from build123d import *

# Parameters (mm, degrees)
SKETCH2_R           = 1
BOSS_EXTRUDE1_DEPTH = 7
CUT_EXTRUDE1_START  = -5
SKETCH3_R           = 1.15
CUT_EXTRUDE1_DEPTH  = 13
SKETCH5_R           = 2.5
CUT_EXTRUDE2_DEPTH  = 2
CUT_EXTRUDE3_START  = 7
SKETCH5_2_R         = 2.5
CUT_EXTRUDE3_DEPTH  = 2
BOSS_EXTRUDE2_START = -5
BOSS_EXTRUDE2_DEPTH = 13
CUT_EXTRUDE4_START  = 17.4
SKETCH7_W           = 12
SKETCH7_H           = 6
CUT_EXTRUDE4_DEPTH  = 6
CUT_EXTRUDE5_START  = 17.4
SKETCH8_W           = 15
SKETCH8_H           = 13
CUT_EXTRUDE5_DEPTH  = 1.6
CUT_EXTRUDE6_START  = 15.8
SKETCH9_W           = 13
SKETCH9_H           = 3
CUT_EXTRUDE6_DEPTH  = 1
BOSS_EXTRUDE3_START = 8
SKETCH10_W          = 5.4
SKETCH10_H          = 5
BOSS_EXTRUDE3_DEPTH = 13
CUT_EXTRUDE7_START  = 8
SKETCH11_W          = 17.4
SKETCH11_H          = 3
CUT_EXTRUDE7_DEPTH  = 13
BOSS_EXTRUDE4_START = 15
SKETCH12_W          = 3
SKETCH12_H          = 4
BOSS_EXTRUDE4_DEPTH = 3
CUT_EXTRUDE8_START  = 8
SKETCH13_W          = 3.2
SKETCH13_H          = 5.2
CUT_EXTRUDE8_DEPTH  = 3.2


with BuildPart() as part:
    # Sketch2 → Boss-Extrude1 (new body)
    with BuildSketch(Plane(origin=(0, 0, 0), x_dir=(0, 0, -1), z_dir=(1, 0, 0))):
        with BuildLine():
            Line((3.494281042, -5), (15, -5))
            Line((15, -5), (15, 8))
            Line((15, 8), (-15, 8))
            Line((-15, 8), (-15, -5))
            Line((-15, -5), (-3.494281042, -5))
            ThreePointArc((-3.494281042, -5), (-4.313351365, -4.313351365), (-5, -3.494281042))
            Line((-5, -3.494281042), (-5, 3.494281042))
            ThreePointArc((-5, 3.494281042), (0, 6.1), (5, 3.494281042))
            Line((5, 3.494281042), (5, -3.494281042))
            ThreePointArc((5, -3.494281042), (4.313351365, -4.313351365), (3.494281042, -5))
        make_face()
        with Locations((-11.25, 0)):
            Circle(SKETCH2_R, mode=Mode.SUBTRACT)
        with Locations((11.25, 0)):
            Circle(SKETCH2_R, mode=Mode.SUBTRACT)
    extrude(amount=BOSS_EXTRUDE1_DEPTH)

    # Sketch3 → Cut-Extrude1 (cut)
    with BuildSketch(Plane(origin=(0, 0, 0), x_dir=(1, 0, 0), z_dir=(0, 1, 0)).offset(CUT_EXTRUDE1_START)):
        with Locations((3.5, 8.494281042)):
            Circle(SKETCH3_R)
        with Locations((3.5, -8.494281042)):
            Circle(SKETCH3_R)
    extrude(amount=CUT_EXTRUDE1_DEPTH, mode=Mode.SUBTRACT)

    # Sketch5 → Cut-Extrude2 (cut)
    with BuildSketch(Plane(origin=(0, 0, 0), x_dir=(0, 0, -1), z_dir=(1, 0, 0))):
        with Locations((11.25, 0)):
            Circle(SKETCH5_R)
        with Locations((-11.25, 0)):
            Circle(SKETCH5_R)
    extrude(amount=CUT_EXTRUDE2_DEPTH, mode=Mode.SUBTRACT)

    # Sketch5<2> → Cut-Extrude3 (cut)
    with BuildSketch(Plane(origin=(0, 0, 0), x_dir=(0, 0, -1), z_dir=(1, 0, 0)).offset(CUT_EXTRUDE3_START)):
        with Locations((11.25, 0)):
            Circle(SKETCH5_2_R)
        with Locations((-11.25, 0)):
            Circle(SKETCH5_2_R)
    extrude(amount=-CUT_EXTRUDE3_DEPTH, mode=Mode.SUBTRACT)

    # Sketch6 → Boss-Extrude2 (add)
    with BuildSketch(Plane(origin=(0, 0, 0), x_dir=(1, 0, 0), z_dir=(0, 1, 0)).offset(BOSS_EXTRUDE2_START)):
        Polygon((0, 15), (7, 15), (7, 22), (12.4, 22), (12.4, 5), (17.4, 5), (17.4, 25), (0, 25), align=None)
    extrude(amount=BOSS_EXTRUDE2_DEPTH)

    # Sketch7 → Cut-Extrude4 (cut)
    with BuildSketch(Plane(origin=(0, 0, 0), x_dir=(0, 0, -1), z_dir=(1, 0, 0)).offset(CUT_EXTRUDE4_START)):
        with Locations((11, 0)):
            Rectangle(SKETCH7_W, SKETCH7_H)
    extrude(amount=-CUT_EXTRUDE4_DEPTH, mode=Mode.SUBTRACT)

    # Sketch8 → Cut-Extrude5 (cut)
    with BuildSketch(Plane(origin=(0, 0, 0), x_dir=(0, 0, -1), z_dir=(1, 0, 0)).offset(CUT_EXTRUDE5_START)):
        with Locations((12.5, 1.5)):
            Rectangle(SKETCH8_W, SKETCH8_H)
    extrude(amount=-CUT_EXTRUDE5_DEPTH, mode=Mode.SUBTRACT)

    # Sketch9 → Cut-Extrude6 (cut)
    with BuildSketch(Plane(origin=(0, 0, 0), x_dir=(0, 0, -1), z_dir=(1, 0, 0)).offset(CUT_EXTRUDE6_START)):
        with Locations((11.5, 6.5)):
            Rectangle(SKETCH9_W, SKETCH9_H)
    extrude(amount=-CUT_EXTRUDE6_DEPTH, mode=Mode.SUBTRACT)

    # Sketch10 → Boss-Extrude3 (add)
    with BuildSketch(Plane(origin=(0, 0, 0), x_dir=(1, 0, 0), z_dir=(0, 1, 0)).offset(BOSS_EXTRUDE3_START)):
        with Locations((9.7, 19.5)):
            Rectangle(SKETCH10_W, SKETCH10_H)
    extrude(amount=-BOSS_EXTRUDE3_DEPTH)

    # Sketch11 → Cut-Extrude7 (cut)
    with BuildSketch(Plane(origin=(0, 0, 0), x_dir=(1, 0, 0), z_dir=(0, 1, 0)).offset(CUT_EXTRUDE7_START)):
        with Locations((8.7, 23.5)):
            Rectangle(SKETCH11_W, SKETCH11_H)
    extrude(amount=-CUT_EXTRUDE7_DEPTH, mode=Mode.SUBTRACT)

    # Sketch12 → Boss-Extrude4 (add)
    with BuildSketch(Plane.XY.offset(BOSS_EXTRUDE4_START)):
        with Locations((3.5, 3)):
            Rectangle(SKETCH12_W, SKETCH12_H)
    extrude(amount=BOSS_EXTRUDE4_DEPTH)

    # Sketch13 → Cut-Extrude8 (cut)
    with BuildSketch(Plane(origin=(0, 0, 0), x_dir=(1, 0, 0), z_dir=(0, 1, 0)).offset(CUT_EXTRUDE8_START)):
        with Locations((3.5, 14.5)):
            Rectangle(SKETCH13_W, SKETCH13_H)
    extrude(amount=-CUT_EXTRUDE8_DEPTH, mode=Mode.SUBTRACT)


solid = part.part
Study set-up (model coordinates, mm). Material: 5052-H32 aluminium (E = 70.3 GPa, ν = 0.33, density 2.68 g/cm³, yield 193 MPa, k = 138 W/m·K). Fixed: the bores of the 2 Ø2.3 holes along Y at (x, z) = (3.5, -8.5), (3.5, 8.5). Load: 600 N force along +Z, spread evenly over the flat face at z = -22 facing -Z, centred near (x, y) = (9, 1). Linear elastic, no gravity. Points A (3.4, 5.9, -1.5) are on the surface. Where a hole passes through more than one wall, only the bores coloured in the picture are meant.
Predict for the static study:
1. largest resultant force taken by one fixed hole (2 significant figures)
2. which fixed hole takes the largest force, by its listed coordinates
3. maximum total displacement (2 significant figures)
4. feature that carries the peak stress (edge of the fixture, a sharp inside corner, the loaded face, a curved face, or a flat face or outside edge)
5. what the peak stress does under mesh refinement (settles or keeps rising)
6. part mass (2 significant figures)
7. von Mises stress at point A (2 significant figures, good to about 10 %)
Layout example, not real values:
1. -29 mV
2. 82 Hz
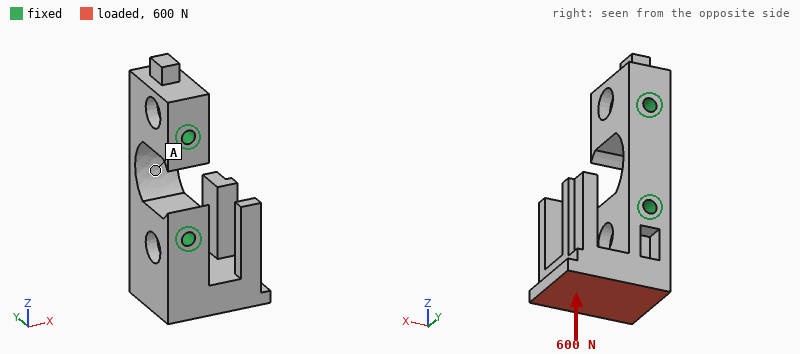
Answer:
1. 590 N
2. (3.5, -8.5)
3. 47 µm
4. edge of the fixture
5. keeps rising
6. 8.6 g
7. 9.0 MPa
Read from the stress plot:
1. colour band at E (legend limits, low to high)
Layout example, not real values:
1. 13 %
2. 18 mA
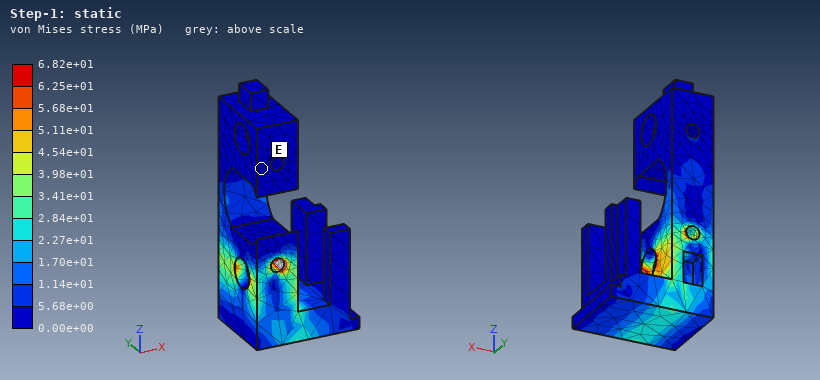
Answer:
1. 0.00e+00 to 5.68e+00 MPa
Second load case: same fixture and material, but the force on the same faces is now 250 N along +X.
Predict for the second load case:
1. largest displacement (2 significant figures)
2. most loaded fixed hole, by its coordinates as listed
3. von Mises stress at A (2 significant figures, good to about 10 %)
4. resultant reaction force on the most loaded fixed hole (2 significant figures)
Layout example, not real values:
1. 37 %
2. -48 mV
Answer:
1. 33 µm
2. (3.5, -8.5)
3. 9.1 MPa
4. 290 N
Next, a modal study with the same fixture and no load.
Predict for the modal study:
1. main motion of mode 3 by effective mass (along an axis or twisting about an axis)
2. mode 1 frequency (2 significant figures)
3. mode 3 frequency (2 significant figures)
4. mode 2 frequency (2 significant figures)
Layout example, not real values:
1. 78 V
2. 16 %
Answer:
1. along X
2. 9000 Hz
3. 12 kHz
4. 9100 Hz
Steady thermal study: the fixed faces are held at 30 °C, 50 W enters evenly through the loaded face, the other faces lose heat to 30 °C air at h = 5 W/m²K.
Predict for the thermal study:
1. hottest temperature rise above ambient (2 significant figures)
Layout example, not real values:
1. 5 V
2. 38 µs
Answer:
1. 77 K
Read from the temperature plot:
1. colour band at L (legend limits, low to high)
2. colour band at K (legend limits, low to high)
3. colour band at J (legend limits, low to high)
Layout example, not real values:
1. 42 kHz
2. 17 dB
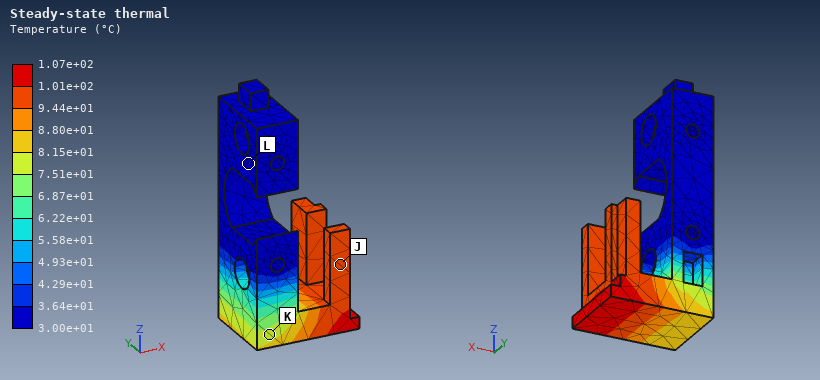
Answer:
1. 3.00e+01 to 3.64e+01 °C
2. 7.51e+01 to 8.15e+01 °C
3. 9.44e+01 to 1.01e+02 °C
